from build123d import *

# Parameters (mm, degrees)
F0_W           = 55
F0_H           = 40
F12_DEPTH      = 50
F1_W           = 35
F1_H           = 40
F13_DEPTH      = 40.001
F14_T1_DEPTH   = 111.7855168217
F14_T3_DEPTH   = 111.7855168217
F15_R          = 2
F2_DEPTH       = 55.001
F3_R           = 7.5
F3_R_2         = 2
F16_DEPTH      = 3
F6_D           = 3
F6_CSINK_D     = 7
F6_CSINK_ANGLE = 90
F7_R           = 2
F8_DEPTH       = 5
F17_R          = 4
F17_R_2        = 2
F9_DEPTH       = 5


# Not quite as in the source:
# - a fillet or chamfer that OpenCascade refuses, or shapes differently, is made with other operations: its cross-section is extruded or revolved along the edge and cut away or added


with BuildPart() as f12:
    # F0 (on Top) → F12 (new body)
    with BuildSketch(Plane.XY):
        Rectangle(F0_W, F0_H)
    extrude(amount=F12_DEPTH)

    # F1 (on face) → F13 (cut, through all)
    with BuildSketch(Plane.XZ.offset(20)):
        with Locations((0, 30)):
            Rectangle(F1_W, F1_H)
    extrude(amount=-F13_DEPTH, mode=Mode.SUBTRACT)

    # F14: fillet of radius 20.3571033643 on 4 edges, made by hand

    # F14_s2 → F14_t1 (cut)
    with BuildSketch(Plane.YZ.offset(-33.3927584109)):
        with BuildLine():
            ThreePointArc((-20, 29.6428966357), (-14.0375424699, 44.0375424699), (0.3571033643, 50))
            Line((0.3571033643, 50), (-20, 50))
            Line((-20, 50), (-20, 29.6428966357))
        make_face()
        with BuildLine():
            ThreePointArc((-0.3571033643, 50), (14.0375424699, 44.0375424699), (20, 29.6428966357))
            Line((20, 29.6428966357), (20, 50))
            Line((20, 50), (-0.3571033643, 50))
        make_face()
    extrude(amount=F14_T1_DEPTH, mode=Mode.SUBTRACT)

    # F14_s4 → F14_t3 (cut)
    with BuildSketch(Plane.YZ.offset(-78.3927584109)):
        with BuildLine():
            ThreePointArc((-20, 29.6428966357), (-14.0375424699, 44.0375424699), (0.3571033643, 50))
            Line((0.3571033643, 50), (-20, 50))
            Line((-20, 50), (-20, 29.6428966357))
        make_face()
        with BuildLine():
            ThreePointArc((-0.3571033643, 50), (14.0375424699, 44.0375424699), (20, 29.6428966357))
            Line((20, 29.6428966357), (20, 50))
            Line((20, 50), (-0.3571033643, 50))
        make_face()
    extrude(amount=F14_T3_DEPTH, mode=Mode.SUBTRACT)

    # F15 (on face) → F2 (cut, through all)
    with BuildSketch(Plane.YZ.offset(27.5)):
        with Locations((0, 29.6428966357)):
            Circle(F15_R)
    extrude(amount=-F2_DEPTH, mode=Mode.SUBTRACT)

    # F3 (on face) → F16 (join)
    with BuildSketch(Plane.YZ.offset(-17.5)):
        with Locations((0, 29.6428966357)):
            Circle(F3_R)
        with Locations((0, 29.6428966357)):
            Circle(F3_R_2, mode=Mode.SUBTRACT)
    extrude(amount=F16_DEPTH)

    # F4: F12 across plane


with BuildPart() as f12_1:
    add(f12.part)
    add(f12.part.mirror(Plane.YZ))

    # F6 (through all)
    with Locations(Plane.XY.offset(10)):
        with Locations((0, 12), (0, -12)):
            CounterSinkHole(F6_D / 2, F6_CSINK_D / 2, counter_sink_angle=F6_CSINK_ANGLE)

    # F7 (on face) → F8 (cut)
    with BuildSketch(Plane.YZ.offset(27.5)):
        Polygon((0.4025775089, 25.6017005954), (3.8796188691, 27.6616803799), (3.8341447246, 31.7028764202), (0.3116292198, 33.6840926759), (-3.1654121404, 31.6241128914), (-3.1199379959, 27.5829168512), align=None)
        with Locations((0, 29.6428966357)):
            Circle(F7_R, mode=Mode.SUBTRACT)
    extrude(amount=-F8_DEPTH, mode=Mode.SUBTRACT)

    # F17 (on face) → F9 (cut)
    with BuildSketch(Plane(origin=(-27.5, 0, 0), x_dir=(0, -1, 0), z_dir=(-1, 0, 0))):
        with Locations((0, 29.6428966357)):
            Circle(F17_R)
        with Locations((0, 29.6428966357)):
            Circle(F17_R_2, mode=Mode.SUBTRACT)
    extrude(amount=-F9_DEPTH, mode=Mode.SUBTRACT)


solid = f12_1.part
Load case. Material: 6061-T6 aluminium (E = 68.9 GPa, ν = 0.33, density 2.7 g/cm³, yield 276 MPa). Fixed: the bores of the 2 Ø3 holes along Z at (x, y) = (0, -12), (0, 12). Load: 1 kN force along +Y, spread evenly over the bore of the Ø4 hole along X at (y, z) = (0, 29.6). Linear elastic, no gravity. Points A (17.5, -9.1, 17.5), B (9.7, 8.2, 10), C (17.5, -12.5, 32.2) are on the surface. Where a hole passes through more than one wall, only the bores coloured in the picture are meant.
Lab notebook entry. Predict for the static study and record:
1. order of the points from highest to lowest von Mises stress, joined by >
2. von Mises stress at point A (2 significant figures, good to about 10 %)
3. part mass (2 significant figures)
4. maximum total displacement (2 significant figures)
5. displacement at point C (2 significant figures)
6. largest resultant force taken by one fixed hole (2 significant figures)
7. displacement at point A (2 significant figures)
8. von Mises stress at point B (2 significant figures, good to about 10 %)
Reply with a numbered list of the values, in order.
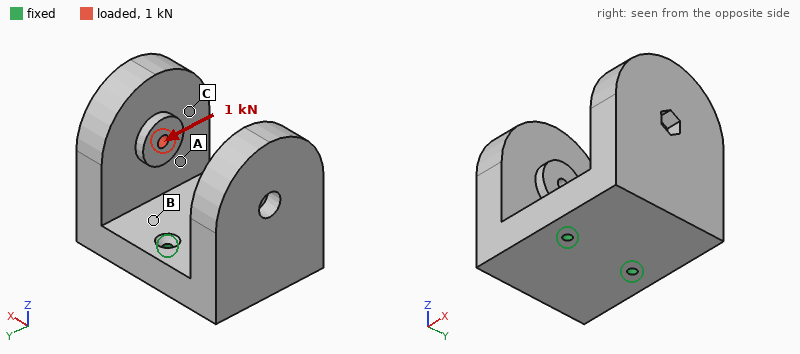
1. B > A > C
2. 15 MPa
3. 140 g
4. 58 µm
5. 40 µm
6. 1.2 kN
7. 21 µm
8. 27 MPa
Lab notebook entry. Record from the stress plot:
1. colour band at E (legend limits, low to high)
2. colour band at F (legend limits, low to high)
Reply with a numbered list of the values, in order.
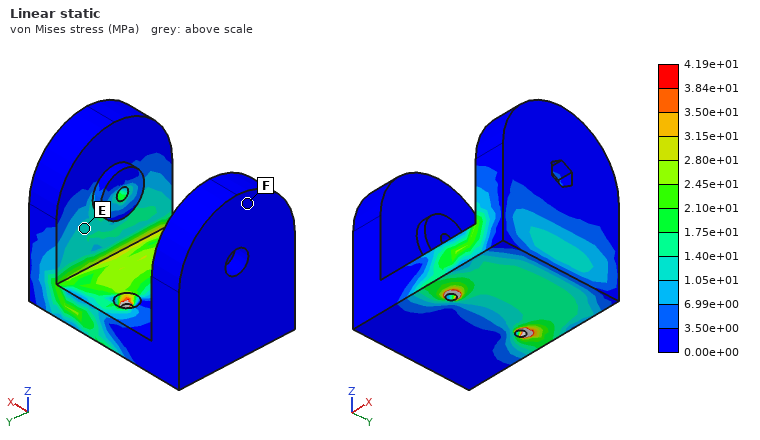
1. 1.05e+01 to 1.40e+01 MPa
2. 0.00e+00 to 3.50e+00 MPa
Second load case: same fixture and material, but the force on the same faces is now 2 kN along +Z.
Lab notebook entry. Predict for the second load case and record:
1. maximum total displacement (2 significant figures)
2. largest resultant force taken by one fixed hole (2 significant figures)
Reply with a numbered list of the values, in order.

1. 0.11 mm
2. 1.0 kN
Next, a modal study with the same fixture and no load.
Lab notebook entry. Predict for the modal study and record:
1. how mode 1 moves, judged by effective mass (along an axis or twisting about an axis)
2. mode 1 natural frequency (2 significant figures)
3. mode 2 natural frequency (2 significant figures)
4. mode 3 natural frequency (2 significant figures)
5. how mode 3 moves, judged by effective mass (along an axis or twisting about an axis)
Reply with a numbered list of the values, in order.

1. along X
2. 2000 Hz
3. 2600 Hz
4. 4000 Hz
5. twisting about Z
